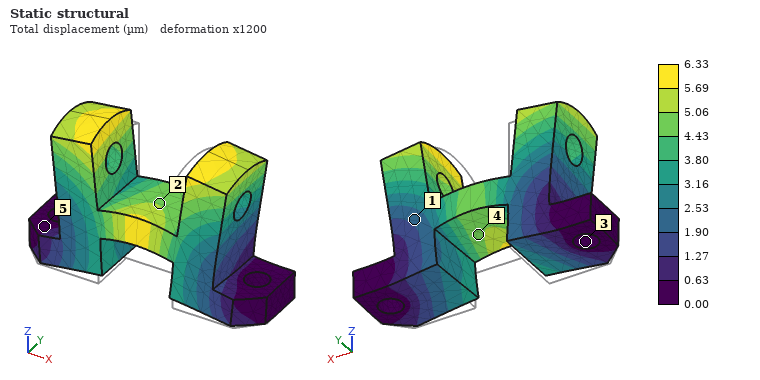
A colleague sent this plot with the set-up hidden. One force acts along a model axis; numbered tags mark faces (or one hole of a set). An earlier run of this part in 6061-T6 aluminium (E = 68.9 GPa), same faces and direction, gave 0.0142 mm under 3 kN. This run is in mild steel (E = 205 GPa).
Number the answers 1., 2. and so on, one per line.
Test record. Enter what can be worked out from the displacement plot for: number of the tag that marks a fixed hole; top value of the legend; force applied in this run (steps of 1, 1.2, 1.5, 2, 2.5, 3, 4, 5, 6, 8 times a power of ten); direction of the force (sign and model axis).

1. 3
2. 6.33 µm
3. 4 kN
4. +Z
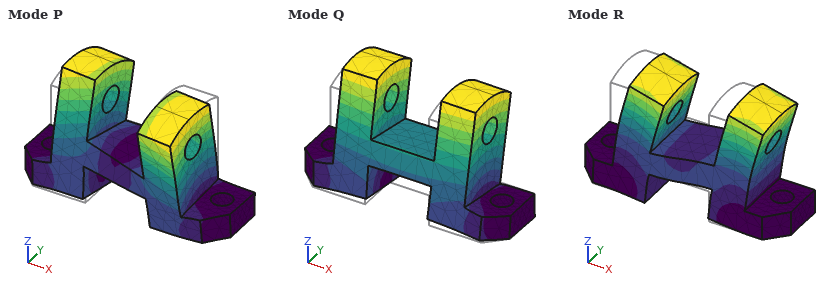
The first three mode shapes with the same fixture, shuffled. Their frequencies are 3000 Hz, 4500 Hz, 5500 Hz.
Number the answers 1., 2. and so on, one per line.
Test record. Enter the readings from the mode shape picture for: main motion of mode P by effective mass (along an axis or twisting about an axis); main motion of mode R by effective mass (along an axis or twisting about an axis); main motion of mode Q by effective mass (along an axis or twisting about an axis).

1. twisting about Z
2. along X
3. along Y
